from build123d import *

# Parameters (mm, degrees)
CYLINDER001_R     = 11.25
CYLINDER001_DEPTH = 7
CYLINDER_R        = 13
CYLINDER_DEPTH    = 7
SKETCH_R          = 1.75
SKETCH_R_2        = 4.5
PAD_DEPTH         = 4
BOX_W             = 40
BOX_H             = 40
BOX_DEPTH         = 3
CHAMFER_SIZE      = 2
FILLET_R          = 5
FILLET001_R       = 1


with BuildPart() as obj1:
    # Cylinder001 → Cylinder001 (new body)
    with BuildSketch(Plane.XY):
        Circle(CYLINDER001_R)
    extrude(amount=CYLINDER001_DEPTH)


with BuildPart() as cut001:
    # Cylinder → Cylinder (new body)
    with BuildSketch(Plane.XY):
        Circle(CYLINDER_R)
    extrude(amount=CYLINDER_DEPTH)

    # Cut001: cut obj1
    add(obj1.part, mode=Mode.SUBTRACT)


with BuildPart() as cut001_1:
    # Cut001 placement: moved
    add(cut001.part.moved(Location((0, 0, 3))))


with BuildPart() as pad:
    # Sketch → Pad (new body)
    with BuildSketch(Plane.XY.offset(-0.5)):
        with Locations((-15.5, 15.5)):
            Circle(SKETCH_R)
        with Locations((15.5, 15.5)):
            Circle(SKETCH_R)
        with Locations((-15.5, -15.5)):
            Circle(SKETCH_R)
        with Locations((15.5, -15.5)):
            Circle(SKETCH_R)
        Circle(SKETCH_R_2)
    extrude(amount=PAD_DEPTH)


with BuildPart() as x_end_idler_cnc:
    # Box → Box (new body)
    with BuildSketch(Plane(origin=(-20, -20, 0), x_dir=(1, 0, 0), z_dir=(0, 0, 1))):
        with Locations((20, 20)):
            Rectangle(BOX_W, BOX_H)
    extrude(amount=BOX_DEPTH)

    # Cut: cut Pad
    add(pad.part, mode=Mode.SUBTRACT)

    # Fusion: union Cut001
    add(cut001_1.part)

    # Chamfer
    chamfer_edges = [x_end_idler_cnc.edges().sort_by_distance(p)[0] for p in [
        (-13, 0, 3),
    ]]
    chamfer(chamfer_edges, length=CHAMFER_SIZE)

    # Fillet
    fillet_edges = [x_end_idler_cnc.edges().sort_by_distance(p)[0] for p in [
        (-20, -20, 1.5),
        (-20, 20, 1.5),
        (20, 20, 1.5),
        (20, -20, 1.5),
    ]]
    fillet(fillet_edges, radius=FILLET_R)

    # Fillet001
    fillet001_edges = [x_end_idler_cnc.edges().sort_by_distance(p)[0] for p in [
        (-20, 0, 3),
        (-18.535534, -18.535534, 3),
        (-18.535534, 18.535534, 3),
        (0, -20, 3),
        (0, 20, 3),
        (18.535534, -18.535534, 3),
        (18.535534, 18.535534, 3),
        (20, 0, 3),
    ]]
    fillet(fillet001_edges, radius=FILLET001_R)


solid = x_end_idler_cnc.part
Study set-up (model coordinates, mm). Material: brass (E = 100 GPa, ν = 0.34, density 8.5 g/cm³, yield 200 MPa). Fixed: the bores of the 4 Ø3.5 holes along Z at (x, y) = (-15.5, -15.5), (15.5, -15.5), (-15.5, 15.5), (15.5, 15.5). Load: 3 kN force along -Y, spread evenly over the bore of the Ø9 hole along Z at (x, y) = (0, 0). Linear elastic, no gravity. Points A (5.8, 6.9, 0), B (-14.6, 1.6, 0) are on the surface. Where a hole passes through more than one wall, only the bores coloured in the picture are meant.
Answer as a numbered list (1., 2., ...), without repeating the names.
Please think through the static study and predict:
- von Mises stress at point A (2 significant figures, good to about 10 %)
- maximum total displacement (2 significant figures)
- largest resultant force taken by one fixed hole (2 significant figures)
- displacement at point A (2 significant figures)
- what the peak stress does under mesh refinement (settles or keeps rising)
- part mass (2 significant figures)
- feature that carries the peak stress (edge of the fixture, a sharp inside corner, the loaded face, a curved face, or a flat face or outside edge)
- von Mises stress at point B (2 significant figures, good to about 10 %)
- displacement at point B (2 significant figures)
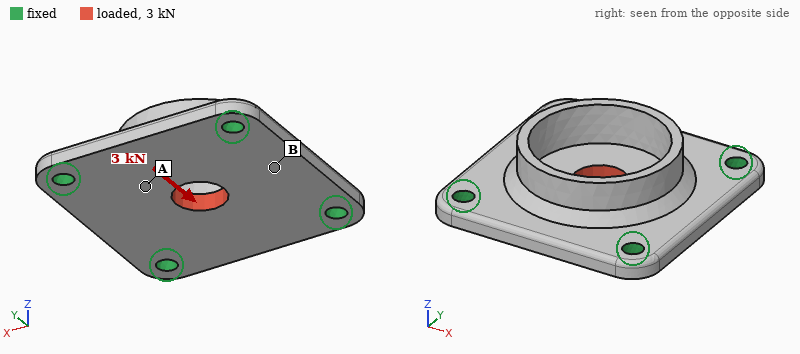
1. 27 MPa
2. 6.8 µm
3. 830 N
4. 4.4 µm
5. keeps rising
6. 47 g
7. edge of the fixture
8. 10 MPa
9. 1.9 µm
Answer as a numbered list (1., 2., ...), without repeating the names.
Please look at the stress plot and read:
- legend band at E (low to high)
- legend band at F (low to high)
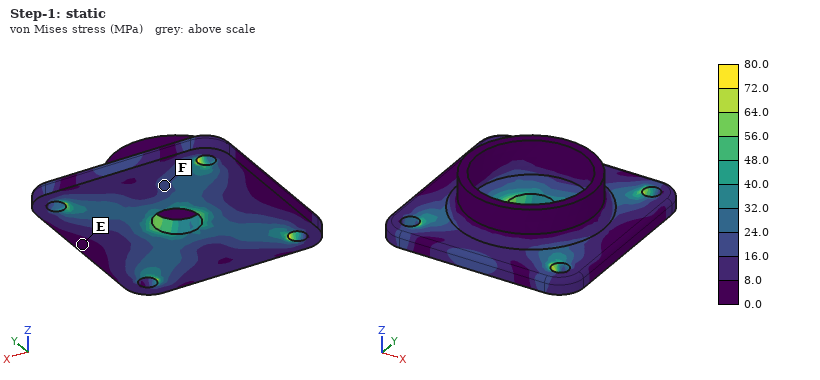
1. 0.0 to 8.0 MPa
2. 16.0 to 24.0 MPa
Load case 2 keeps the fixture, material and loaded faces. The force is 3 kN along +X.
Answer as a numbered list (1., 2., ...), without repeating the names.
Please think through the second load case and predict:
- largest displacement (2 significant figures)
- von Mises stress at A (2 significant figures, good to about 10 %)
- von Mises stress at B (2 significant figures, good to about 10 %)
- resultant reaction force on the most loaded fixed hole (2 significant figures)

1. 6.8 µm
2. 26 MPa
3. 9.7 MPa
4. 830 N
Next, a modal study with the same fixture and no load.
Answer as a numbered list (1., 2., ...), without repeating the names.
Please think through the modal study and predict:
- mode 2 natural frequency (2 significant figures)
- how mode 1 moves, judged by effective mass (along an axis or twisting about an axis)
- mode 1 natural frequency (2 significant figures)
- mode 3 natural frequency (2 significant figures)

1. 13 kHz
2. along Z
3. 9300 Hz
4. 13 kHz
